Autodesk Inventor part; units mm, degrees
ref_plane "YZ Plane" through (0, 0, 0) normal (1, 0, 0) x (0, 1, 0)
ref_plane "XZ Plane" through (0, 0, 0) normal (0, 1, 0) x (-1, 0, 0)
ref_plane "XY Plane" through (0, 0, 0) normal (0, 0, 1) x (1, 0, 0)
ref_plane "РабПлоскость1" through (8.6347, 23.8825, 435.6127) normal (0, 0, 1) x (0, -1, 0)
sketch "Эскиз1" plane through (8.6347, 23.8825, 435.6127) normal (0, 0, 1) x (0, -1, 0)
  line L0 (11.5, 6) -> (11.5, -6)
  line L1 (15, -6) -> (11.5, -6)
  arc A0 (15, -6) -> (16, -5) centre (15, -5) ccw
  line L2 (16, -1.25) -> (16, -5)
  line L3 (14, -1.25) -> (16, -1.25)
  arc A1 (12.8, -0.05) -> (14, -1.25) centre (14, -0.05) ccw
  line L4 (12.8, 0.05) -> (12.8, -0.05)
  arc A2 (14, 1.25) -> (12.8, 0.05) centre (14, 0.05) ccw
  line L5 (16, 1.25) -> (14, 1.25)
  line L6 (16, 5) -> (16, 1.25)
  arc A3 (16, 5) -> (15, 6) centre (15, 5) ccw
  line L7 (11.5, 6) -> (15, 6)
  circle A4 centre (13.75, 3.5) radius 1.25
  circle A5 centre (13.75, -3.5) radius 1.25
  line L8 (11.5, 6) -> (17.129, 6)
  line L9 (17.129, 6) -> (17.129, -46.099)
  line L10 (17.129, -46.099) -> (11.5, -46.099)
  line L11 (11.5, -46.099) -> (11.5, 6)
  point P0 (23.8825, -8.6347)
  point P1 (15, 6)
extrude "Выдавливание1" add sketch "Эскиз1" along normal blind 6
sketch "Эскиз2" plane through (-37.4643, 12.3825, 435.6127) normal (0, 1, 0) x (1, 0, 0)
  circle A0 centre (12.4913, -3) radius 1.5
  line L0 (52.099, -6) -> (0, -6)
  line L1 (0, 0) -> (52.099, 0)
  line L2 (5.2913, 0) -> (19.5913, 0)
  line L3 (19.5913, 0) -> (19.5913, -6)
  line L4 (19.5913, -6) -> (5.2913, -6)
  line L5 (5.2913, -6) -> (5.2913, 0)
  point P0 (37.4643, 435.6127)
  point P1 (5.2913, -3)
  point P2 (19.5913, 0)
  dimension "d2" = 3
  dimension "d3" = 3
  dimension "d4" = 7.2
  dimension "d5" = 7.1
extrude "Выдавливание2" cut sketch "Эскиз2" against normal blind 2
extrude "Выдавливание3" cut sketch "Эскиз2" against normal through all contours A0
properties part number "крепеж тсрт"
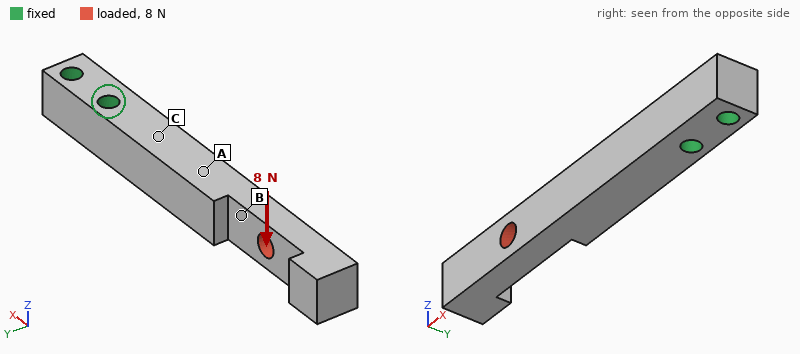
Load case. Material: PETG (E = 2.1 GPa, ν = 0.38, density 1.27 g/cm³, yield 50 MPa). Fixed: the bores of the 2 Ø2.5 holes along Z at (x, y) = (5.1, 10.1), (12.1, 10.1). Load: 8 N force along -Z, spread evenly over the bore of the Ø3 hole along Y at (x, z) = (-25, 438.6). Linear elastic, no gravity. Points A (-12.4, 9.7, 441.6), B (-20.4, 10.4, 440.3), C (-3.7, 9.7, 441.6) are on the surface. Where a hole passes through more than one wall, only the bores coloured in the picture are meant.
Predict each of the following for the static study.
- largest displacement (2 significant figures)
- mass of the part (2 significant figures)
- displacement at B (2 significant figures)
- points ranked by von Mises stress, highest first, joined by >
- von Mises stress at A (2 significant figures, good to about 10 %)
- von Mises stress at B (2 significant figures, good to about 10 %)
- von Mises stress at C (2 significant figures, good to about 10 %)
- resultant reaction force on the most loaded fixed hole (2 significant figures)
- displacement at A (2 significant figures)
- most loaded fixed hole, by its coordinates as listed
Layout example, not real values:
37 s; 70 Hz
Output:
0.57 mm; 1.9 g; 0.26 mm; C > A > B; 3.0 MPa; 1.2 MPa; 5.1 MPa; 10 N; 0.14 mm; (5.1, 10.1)
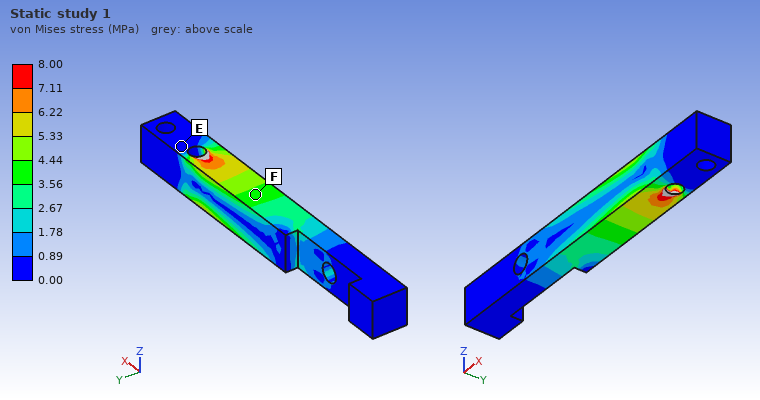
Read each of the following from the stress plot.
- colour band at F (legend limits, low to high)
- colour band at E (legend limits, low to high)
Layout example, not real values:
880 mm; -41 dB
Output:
3.56 to 4.44 MPa; 0.00 to 0.89 MPa
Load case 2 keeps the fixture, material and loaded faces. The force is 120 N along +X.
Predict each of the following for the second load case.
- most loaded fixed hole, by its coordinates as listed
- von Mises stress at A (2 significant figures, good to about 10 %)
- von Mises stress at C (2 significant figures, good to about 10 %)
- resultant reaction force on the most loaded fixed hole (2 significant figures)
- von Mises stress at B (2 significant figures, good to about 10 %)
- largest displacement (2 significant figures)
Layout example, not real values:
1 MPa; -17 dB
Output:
(5.1, 10.1); 3.4 MPa; 3.3 MPa; 110 N; 5.5 MPa; 0.51 mm
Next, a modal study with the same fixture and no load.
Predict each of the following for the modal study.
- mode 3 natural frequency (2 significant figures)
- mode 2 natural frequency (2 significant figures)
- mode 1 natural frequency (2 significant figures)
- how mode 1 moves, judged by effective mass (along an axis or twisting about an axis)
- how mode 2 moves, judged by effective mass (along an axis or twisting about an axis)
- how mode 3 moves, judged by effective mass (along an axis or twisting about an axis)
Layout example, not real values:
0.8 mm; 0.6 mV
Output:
2600 Hz; 760 Hz; 640 Hz; along Y; along Z; along Y
